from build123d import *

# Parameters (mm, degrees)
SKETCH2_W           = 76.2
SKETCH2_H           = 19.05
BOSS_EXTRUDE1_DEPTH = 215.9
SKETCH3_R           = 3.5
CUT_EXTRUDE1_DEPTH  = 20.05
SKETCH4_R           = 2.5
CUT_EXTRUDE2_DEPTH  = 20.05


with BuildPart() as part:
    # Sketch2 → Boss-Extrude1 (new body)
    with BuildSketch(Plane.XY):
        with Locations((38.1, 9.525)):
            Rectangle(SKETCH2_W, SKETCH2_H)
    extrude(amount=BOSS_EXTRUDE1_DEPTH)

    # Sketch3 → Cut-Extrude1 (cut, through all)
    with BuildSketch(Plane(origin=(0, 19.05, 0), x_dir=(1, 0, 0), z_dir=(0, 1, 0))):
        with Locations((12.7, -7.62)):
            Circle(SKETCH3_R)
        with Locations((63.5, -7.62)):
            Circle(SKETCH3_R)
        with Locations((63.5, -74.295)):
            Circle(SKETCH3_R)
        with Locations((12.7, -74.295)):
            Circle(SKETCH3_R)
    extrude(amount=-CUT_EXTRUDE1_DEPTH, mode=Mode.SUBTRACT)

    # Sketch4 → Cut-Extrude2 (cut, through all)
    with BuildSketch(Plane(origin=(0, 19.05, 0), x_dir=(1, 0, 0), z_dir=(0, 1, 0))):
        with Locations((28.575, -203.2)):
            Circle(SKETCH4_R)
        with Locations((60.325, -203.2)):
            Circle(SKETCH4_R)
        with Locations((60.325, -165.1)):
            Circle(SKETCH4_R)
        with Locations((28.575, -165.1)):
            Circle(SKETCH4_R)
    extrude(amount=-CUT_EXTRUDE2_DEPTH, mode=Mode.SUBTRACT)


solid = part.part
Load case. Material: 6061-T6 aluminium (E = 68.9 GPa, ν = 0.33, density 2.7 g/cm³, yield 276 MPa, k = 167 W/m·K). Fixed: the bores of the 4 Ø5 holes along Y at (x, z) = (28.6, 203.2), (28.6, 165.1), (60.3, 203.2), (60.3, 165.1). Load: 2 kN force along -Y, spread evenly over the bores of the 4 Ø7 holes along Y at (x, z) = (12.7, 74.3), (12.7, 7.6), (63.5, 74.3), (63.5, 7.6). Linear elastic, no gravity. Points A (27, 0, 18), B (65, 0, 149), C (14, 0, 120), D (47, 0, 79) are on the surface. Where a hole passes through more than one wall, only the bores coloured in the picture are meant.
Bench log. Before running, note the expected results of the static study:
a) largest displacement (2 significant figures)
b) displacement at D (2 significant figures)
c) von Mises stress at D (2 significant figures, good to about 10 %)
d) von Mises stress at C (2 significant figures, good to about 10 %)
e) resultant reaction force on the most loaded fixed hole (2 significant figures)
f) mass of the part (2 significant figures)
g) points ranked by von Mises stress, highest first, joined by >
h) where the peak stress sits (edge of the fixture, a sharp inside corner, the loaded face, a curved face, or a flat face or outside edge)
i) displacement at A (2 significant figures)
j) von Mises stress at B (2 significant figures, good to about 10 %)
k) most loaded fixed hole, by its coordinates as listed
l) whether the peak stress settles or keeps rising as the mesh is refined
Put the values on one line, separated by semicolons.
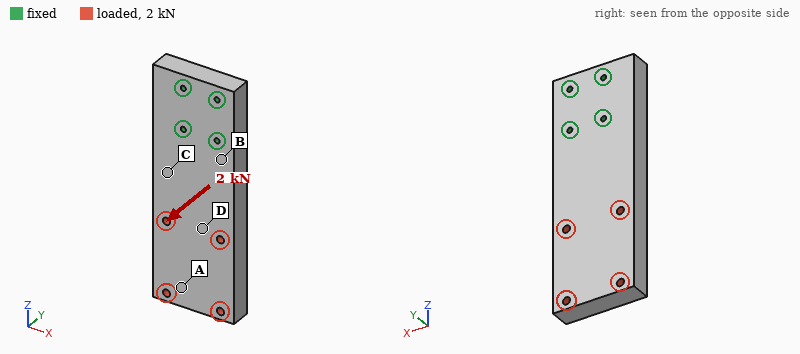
0.71 mm; 0.27 mm; 18 MPa; 33 MPa; 3.0 kN; 830 g; B > C > D > A; edge of the fixture; 0.60 mm; 48 MPa; (28.6, 165.1); keeps rising
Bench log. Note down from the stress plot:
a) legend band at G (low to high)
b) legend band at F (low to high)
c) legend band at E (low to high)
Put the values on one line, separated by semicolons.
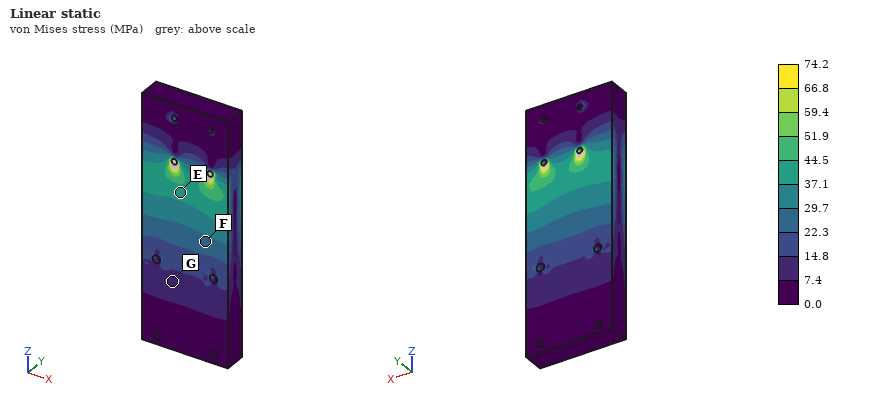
7.4 to 14.8 MPa; 22.3 to 29.7 MPa; 37.1 to 44.5 MPa
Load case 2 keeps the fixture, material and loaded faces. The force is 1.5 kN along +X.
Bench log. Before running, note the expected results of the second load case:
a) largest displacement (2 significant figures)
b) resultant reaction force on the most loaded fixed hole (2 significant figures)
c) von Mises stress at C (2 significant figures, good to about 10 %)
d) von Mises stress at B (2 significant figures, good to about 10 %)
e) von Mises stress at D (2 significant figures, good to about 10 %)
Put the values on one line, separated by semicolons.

51 µm; 3.5 kN; 4.3 MPa; 7.3 MPa; 2.4 MPa
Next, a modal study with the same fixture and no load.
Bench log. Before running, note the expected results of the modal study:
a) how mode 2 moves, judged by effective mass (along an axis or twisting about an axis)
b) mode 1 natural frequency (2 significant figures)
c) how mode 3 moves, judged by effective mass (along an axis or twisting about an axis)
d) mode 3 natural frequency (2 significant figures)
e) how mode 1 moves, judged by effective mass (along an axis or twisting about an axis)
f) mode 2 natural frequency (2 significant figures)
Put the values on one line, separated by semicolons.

along X; 550 Hz; twisting about Z; 2200 Hz; along Y; 1700 Hz
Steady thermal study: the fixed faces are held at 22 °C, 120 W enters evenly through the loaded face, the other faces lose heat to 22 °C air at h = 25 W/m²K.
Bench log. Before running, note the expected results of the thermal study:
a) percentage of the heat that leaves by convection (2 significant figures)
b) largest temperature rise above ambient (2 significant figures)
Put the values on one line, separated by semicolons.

22 %; 55 K
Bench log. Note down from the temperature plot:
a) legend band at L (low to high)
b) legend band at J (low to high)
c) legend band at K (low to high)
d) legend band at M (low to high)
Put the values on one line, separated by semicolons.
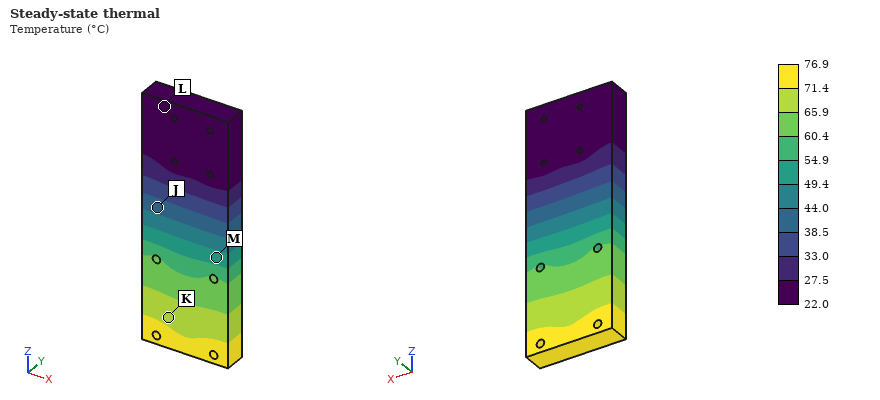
22.0 to 27.5 °C; 38.5 to 44.0 °C; 65.9 to 71.4 °C; 49.4 to 54.9 °C
